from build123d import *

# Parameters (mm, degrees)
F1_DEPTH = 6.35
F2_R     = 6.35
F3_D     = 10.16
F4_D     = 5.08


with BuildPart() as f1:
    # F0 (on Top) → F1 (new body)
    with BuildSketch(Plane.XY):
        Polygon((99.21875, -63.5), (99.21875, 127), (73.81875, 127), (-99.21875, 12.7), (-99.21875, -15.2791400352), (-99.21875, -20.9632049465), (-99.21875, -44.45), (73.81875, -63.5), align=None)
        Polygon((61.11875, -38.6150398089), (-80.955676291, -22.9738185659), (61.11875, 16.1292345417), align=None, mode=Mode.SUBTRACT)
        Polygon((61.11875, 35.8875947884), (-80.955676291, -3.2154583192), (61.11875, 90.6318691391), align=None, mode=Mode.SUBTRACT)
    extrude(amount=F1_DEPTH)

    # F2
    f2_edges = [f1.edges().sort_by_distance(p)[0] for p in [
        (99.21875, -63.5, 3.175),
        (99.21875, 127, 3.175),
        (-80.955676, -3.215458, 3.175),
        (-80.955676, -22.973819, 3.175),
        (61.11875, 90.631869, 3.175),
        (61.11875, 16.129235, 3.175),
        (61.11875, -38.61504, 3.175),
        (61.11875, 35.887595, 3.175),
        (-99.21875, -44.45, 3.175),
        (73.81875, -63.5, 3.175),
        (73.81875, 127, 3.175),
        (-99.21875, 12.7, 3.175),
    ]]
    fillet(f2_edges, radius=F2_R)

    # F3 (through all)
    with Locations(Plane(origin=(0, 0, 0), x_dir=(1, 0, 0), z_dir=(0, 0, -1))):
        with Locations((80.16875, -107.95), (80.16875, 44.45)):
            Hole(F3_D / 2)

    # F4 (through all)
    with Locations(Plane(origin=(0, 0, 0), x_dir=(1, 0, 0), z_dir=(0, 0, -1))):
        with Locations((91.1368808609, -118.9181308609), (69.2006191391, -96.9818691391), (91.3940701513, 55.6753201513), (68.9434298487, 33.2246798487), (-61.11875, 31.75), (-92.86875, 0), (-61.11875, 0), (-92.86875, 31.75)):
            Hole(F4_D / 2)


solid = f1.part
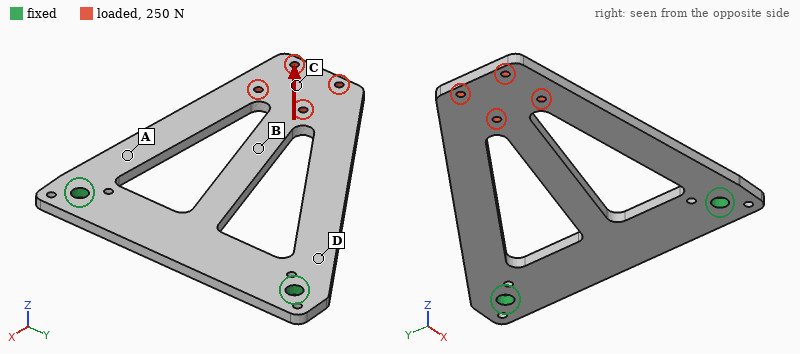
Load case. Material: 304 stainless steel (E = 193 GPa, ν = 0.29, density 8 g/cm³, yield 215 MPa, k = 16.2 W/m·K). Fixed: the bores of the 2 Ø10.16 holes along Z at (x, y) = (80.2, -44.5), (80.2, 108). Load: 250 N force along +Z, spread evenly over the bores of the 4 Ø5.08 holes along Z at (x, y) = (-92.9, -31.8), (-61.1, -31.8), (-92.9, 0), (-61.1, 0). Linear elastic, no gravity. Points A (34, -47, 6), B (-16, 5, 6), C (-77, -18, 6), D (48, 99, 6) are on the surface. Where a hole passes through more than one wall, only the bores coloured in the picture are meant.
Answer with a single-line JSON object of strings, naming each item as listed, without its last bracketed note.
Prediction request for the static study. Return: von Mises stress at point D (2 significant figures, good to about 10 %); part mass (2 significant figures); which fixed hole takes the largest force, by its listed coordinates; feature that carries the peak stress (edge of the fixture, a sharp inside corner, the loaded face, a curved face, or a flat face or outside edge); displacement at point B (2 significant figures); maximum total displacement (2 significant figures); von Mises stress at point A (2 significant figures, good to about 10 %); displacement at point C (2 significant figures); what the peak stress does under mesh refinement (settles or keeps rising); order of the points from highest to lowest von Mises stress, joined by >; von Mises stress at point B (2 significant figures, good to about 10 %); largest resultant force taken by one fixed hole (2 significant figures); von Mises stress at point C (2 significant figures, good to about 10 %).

{"von Mises stress at point D": "55 MPa", "part mass": "940 g", "which fixed hole takes the largest force, by its listed coordinates": "(80.2, -44.5)", "feature that carries the peak stress": "edge of the fixture", "displacement at point B": "0.54 mm", "maximum total displacement": "1.5 mm", "von Mises stress at point A": "75 MPa", "displacement at point C": "1.2 mm", "what the peak stress does under mesh refinement": "keeps rising", "order of the points from highest to lowest von Mises stress, joined by >": "A > D > B > C", "von Mises stress at point B": "33 MPa", "largest resultant force taken by one fixed hole": "190 N", "von Mises stress at point C": "13 MPa"}
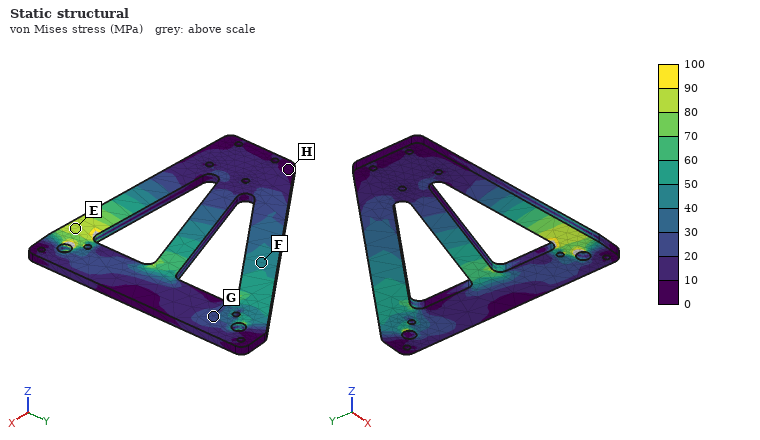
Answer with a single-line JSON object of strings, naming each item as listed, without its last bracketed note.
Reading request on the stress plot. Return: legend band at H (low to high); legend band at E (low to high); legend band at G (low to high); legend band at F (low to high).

{"legend band at H": "0 to 10 MPa", "legend band at E": "80 to 90 MPa", "legend band at G": "20 to 30 MPa", "legend band at F": "40 to 50 MPa"}
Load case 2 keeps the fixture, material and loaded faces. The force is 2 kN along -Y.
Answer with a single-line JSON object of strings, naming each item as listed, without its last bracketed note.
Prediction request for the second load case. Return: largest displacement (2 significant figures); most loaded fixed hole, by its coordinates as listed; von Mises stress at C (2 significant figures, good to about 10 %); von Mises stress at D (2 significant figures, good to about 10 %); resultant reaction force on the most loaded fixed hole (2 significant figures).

{"largest displacement": "48 µm", "most loaded fixed hole, by its coordinates as listed": "(80.2, 108)", "von Mises stress at C": "7.9 MPa", "von Mises stress at D": "18 MPa", "resultant reaction force on the most loaded fixed hole": "2.3 kN"}
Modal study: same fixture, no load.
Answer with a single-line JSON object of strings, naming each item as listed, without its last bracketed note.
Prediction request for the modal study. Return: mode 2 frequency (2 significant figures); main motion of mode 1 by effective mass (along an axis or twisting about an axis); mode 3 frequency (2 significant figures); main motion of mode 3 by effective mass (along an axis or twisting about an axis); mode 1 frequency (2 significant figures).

{"mode 2 frequency": "620 Hz", "main motion of mode 1 by effective mass": "along Z", "mode 3 frequency": "920 Hz", "main motion of mode 3 by effective mass": "along Z", "mode 1 frequency": "150 Hz"}
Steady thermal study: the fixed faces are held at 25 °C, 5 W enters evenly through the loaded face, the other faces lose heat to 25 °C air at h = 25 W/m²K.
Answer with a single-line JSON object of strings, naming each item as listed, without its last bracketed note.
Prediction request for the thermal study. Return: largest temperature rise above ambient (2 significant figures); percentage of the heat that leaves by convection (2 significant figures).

{"largest temperature rise above ambient": "23 K", "percentage of the heat that leaves by convection": "98 %"}
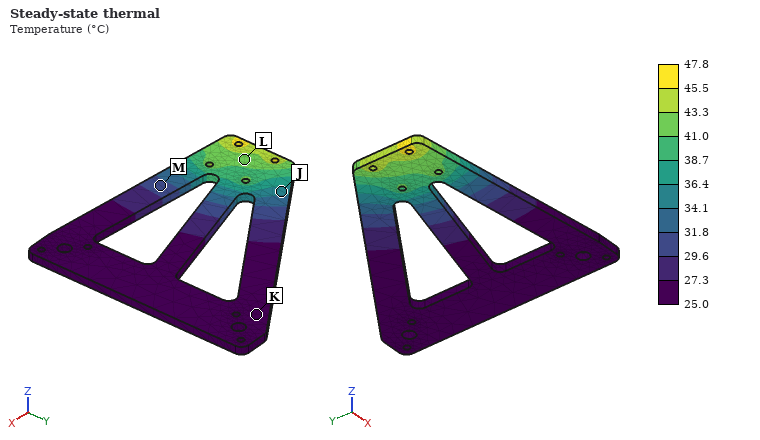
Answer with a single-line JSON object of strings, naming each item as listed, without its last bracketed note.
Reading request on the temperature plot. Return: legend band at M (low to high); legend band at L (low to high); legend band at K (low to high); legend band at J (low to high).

{"legend band at M": "29.6 to 31.8 °C", "legend band at L": "41.0 to 43.3 °C", "legend band at K": "25.0 to 27.3 °C", "legend band at J": "34.1 to 36.4 °C"}
